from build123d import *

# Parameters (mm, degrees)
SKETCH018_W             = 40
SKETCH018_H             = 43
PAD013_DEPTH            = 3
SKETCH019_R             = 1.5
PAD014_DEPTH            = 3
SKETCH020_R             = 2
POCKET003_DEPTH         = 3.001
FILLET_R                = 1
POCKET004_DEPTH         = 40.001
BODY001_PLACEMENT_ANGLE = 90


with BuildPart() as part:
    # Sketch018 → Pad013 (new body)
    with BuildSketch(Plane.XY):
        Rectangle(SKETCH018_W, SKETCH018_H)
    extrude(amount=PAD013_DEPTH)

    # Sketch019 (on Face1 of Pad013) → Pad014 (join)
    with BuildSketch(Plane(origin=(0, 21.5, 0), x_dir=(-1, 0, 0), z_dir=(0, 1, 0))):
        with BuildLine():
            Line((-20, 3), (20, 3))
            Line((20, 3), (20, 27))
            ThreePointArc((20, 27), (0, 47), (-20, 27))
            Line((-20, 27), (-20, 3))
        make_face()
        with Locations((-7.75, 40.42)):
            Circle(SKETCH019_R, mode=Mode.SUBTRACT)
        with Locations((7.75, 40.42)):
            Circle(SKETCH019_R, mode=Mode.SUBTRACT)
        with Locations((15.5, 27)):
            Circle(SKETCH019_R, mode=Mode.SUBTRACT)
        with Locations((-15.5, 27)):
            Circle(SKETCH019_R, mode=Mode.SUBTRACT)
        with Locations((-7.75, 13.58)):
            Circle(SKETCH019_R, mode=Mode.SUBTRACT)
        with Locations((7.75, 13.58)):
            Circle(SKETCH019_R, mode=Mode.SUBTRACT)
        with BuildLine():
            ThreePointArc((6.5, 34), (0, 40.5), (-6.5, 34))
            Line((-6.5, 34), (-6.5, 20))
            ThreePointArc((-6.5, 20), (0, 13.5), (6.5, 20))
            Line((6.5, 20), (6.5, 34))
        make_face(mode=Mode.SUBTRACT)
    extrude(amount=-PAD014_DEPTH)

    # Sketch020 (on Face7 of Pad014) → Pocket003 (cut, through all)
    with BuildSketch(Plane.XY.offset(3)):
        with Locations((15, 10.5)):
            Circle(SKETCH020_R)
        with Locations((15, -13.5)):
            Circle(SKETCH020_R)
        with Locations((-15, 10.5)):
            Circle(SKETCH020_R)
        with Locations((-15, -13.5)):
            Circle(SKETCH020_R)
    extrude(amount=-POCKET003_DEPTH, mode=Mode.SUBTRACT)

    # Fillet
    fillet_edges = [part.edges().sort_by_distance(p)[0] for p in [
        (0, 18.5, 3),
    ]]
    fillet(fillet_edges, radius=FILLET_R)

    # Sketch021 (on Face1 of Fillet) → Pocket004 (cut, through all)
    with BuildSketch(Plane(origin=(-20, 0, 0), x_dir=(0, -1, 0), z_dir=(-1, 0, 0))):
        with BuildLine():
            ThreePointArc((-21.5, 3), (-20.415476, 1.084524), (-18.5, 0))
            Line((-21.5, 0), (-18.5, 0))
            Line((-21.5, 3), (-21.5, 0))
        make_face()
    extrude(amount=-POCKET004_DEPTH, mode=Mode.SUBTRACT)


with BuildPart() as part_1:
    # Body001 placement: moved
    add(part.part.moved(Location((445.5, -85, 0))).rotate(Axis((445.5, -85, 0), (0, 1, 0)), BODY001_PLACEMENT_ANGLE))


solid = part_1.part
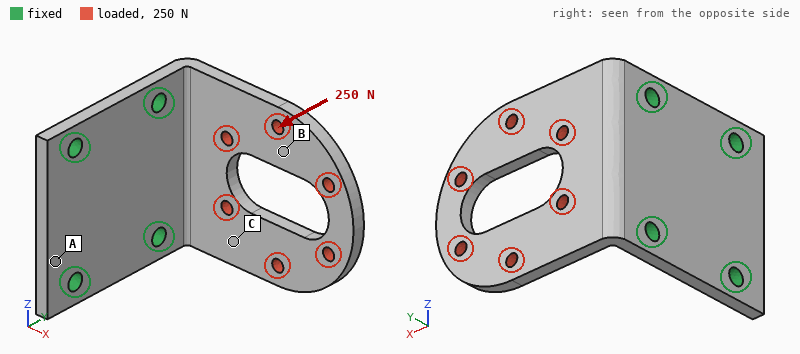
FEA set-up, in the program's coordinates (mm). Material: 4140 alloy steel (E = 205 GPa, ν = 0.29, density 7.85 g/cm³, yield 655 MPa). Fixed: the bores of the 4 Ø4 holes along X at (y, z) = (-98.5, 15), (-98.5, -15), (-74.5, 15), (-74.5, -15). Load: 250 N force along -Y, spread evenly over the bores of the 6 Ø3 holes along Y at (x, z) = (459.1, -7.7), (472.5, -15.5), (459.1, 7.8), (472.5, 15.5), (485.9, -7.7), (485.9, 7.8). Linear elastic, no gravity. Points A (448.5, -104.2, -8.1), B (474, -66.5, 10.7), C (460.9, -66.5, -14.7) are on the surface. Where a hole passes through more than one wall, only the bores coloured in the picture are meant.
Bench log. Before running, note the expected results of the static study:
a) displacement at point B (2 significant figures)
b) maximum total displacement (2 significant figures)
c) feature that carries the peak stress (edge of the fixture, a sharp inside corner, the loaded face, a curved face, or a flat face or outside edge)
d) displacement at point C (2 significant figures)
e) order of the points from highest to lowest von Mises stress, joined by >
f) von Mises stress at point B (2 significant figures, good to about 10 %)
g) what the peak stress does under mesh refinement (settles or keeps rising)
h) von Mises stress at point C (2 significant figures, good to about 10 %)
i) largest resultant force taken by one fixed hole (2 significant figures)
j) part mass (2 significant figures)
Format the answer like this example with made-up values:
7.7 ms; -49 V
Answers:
0.17 mm; 0.34 mm; edge of the fixture; 0.066 mm; C > B > A; 32 MPa; keeps rising; 70 MPa; 92 N; 68 g
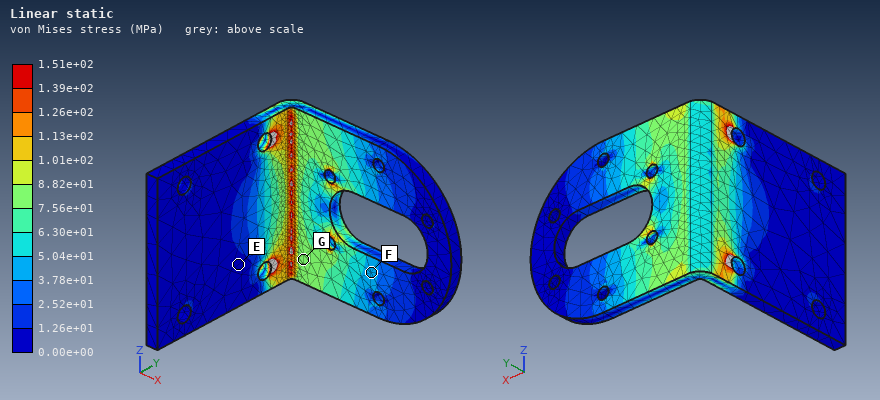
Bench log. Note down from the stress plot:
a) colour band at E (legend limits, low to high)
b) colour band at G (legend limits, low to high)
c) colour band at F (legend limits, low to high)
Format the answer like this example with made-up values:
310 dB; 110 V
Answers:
0.00e+00 to 1.26e+01 MPa; 7.56e+01 to 8.82e+01 MPa; 3.78e+01 to 5.04e+01 MPa
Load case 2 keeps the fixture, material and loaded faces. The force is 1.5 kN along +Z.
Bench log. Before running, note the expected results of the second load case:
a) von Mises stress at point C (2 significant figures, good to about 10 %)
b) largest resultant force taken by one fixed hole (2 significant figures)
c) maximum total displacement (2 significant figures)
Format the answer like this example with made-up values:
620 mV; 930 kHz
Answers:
62 MPa; 1.5 kN; 0.12 mm
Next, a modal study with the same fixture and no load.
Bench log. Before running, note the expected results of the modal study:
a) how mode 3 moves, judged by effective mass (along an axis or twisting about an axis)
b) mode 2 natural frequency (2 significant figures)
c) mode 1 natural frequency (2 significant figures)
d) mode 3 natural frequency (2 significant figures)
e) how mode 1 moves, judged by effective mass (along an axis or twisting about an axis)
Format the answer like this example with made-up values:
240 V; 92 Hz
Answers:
along Z; 3100 Hz; 1200 Hz; 4900 Hz; along Y
